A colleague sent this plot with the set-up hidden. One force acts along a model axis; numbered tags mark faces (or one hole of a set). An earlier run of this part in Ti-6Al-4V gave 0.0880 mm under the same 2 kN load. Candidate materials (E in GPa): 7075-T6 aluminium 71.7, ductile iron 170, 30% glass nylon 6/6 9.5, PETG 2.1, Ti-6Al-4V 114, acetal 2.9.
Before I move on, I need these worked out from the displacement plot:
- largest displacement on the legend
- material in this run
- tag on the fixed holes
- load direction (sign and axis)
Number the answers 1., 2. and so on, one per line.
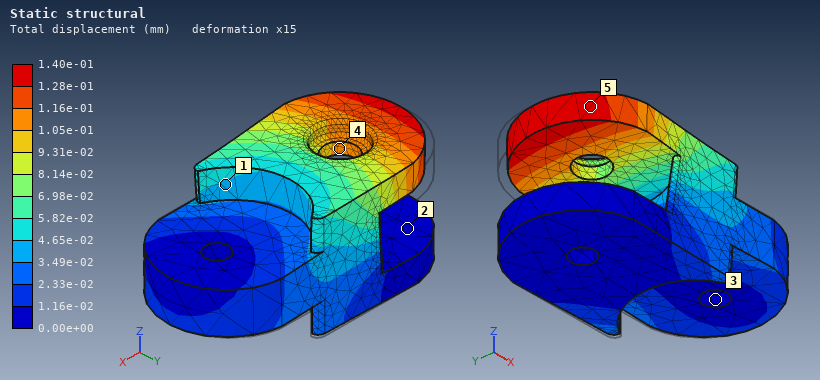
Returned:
1. 1.40e-01 mm
2. 7075-T6 aluminium
3. 3
4. -Y
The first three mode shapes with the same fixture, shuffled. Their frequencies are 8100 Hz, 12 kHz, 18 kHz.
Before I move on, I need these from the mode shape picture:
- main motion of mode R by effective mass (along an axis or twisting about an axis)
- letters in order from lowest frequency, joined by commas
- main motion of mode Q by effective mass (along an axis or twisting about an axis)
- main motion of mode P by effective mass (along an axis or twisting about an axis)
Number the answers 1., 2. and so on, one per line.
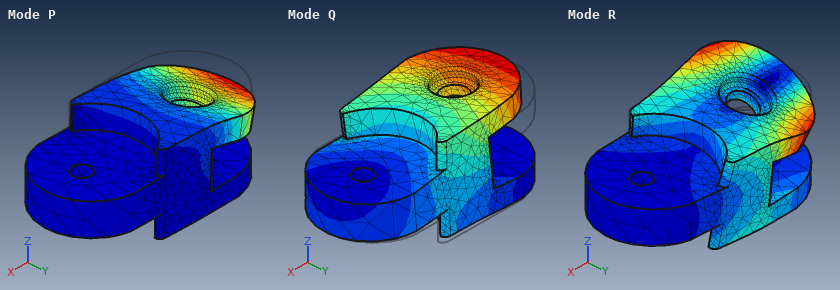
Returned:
1. twisting about X
2. P, Q, R
3. along Y
4. along Z
